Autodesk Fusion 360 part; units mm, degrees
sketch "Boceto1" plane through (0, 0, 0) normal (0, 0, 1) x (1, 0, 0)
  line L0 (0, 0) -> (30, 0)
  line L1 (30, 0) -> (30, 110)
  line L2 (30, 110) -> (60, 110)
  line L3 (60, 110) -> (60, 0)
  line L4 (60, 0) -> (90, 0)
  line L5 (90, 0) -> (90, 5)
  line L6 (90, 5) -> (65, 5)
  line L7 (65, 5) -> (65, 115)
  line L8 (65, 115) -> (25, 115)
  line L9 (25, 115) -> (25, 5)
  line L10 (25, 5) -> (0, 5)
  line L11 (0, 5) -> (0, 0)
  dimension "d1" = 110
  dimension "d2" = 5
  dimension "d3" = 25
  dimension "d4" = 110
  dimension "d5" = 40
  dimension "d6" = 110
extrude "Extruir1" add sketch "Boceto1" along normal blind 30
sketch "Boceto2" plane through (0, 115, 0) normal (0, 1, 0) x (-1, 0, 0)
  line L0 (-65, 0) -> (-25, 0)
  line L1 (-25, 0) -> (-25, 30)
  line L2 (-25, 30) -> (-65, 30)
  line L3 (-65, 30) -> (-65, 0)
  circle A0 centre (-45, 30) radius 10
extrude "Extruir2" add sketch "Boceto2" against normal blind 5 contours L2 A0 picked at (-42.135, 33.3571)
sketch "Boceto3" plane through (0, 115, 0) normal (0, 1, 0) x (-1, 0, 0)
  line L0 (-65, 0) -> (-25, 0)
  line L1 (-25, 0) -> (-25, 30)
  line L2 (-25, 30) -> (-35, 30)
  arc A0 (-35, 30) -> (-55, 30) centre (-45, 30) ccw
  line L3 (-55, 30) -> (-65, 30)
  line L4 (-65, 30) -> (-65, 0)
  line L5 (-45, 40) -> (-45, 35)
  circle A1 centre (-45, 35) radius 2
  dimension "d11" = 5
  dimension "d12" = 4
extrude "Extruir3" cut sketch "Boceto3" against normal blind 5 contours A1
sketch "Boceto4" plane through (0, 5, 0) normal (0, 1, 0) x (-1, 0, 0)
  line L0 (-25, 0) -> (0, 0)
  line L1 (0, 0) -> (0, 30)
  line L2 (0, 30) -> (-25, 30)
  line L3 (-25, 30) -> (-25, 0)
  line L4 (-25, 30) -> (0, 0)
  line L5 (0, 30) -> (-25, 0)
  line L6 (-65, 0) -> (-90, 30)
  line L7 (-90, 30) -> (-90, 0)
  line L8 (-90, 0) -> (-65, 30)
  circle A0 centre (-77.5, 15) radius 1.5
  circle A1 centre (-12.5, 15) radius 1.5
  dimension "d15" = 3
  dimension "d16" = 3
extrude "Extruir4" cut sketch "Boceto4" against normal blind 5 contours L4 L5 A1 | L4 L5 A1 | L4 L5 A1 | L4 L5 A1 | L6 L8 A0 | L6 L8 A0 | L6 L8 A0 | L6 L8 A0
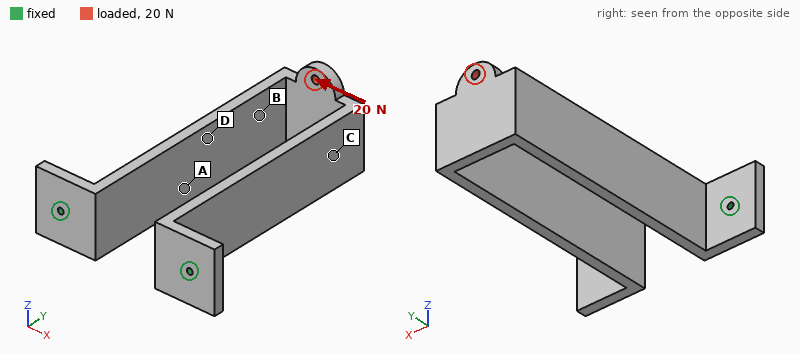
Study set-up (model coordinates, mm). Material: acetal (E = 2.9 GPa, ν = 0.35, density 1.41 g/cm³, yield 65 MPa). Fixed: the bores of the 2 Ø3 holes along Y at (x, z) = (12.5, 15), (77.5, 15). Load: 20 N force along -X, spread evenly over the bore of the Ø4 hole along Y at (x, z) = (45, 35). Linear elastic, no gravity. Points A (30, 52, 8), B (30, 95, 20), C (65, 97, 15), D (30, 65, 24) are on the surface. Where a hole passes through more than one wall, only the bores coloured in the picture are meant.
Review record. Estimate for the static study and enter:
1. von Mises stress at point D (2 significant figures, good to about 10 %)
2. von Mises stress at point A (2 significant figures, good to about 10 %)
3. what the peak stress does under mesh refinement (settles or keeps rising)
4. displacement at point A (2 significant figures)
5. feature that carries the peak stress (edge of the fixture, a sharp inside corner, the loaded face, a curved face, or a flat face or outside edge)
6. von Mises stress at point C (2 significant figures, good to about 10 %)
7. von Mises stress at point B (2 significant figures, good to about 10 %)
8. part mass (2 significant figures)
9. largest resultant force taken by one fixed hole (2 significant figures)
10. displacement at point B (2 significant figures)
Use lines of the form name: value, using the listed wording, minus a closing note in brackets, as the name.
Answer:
von Mises stress at point D: 1.7 MPa
von Mises stress at point A: 0.82 MPa
what the peak stress does under mesh refinement: keeps rising
displacement at point A: 0.61 mm
feature that carries the peak stress: edge of the fixture
von Mises stress at point C: 2.9 MPa
von Mises stress at point B: 3.5 MPa
part mass: 66 g
largest resultant force taken by one fixed hole: 34 N
displacement at point B: 1.4 mm
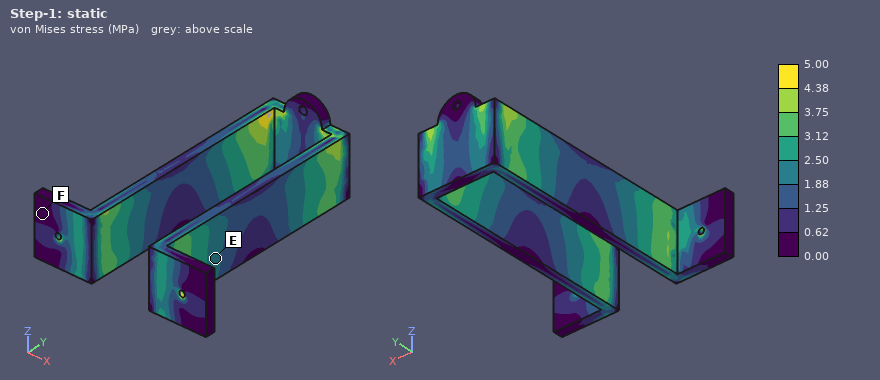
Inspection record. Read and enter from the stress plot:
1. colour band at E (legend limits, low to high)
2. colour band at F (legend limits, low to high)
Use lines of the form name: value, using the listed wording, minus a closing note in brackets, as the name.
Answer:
colour band at E: 1.88 to 2.50 MPa
colour band at F: 0.00 to 0.62 MPa
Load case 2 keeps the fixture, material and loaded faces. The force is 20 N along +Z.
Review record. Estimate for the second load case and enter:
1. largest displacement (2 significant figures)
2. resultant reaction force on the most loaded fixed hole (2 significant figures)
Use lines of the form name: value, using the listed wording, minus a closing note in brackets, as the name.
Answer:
largest displacement: 1.7 mm
resultant reaction force on the most loaded fixed hole: 10 N
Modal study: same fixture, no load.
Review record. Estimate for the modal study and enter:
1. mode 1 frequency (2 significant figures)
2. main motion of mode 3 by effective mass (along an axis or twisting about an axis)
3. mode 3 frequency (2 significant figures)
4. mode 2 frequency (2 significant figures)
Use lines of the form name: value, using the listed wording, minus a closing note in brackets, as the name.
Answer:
mode 1 frequency: 110 Hz
main motion of mode 3 by effective mass: twisting about Y
mode 3 frequency: 320 Hz
mode 2 frequency: 110 Hz
